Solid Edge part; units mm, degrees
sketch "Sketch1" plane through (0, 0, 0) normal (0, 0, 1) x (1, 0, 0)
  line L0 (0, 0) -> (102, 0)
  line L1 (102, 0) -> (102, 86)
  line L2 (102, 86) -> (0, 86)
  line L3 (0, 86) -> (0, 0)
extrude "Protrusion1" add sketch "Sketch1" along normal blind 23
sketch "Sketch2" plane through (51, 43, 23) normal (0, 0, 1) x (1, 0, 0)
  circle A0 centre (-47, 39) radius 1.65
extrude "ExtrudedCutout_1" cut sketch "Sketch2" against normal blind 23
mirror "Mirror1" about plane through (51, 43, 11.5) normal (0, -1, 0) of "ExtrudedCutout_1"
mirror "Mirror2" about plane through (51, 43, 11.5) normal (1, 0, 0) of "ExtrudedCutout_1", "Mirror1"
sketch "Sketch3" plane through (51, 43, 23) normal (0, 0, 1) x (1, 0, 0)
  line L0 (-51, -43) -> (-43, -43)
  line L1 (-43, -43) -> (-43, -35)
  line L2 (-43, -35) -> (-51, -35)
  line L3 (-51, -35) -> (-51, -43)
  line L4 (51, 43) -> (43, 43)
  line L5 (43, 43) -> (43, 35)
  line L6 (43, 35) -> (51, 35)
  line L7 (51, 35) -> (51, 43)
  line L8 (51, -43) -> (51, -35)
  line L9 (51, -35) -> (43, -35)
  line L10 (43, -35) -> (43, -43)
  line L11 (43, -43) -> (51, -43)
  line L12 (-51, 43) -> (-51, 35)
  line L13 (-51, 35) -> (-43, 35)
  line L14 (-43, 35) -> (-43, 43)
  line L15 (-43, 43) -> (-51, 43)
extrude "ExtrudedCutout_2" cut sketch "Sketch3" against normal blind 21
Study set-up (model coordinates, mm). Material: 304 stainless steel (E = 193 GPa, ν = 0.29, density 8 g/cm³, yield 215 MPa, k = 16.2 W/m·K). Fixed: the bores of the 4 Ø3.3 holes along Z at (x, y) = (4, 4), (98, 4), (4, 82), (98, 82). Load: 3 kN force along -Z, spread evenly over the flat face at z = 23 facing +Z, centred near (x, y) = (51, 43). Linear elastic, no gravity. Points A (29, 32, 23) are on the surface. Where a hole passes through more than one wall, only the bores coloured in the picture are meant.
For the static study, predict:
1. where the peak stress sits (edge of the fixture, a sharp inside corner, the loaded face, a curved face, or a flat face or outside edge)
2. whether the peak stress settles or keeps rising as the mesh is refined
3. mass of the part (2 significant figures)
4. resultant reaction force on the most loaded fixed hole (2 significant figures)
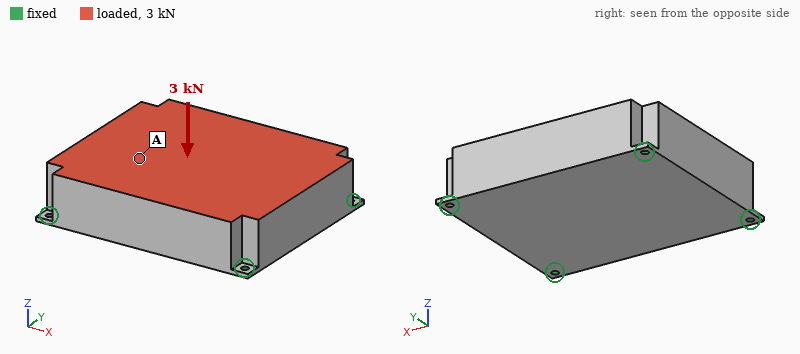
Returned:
edge of the fixture
keeps rising
1.6 kg
880 N
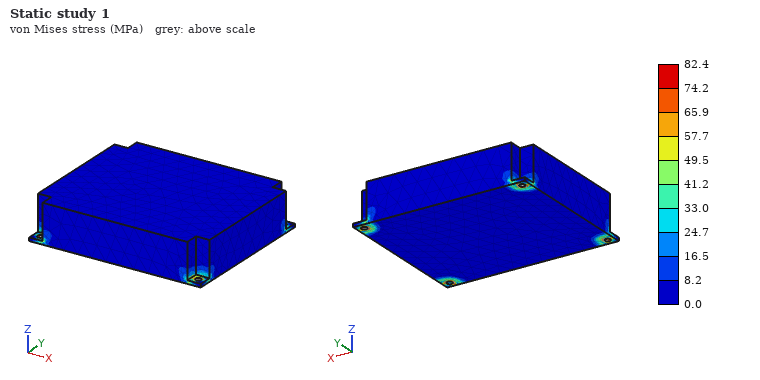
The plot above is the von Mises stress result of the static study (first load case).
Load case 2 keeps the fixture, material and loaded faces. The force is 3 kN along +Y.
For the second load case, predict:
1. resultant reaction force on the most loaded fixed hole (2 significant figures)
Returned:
910 N
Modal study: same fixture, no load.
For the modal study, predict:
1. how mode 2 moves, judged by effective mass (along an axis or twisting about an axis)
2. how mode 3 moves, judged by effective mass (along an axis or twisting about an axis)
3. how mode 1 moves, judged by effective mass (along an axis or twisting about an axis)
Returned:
along Y
along X
along Z
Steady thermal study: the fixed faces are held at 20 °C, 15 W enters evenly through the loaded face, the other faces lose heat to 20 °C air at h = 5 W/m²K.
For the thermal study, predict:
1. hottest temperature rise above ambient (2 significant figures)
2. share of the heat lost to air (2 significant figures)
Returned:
44 K
23 %
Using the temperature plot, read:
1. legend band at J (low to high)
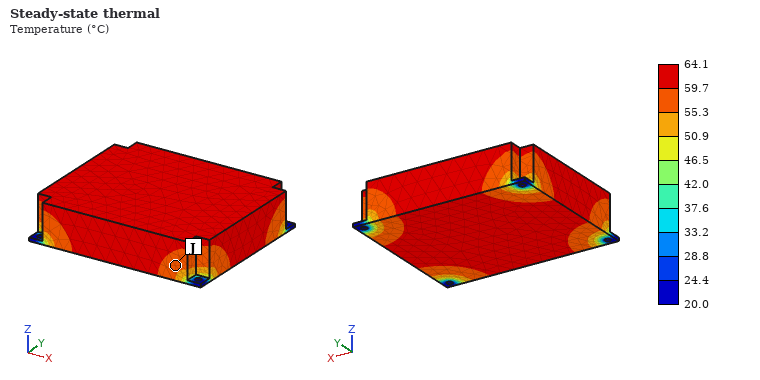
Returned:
55.3 to 59.7 °C
